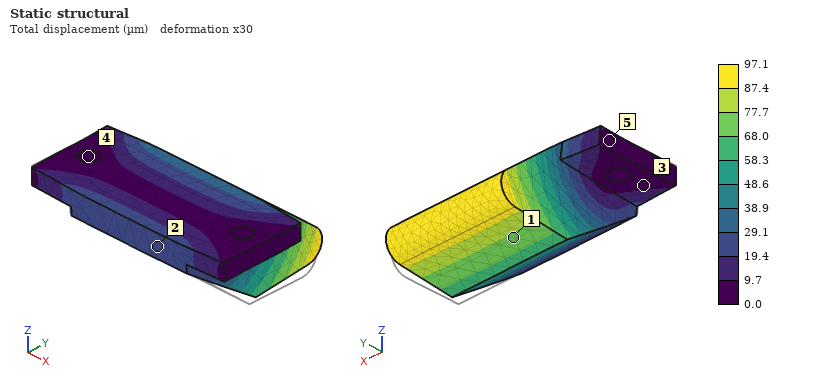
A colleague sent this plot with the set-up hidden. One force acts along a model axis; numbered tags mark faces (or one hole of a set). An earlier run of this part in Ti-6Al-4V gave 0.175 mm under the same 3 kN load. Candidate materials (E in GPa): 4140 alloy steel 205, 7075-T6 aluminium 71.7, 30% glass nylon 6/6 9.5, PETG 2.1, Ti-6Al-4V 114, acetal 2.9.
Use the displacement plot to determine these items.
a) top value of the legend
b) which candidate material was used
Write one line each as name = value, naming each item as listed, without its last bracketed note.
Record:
top value of the legend = 97.1 µm
which candidate material was used = 4140 alloy steel
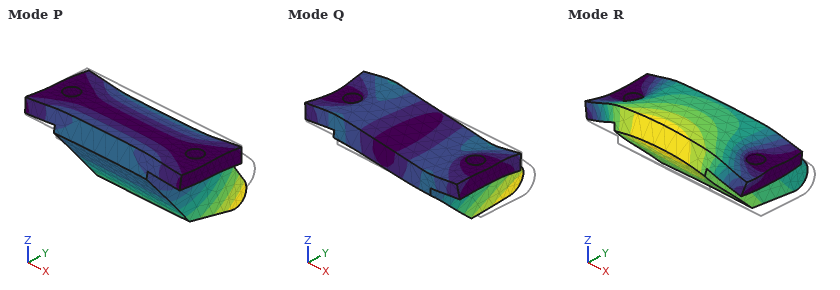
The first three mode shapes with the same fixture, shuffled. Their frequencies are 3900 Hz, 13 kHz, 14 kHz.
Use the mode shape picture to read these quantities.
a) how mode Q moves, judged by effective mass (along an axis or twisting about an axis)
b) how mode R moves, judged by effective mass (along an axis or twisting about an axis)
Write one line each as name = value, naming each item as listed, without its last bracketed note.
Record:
how mode Q moves, judged by effective mass = along X
how mode R moves, judged by effective mass = along Z
